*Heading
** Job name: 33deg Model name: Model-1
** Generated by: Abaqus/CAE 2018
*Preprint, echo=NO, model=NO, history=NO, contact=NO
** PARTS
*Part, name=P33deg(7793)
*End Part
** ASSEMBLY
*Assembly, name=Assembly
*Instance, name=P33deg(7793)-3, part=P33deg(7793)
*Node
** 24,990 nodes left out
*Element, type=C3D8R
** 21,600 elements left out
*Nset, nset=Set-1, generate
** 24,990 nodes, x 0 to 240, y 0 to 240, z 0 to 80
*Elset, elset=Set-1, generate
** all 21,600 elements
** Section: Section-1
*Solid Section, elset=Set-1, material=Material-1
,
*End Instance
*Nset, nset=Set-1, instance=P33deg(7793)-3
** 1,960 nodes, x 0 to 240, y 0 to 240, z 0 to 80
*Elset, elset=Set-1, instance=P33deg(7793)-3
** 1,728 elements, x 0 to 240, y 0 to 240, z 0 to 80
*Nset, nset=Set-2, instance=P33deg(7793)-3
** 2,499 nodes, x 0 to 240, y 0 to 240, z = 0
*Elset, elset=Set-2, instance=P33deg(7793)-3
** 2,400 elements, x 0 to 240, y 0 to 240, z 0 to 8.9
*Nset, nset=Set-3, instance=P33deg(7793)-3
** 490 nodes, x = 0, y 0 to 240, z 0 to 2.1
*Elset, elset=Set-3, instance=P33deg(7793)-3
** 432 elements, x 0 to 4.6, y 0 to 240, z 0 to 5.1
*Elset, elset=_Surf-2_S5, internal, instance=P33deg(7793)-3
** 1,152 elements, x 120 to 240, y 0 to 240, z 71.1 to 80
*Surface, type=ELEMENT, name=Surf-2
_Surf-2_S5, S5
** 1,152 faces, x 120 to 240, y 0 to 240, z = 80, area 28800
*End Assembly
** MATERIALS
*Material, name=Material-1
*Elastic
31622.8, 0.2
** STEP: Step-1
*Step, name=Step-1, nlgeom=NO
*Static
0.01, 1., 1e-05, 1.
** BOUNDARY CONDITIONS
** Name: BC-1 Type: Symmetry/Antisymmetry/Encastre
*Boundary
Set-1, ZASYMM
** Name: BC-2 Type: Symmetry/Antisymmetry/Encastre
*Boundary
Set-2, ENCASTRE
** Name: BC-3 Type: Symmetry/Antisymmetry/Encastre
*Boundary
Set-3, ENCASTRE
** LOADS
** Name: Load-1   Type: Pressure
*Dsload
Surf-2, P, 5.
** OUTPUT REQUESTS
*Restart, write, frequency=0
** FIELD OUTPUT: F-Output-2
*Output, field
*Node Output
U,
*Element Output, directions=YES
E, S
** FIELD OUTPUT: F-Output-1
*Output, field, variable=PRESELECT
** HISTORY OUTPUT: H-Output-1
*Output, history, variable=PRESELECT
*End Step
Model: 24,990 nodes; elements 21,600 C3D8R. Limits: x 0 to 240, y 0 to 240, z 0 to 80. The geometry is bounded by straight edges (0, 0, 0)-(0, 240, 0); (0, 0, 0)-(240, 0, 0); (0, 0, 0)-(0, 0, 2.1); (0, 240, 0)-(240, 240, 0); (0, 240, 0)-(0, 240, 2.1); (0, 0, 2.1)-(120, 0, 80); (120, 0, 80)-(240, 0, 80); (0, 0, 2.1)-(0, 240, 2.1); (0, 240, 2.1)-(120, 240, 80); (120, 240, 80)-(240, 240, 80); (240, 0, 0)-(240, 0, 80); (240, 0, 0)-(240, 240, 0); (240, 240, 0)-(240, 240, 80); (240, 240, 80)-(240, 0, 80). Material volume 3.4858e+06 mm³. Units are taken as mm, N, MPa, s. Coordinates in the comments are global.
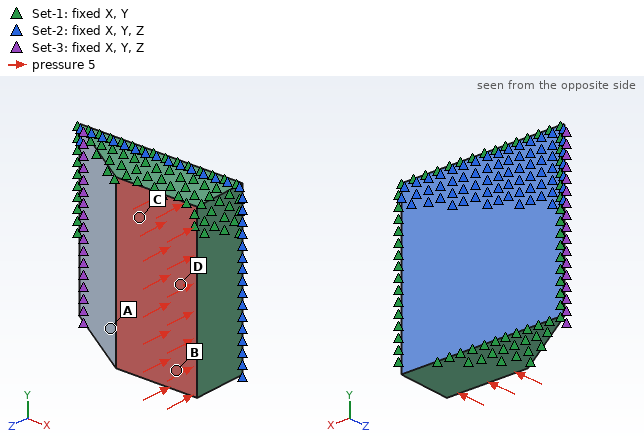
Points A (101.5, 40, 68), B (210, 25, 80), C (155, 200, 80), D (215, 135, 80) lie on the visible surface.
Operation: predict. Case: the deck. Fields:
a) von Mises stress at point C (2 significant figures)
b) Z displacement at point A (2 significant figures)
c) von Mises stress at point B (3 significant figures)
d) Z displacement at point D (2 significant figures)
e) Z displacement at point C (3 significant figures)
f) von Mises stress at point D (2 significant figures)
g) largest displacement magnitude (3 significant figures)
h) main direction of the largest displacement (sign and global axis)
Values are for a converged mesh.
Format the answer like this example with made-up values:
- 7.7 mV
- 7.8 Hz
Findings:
- 3.2 MPa
- -0.0019 mm
- 3.65 MPa
- -0.011 mm
- -0.0105 mm
- 3.6 MPa
- 0.0115 mm
- -Z
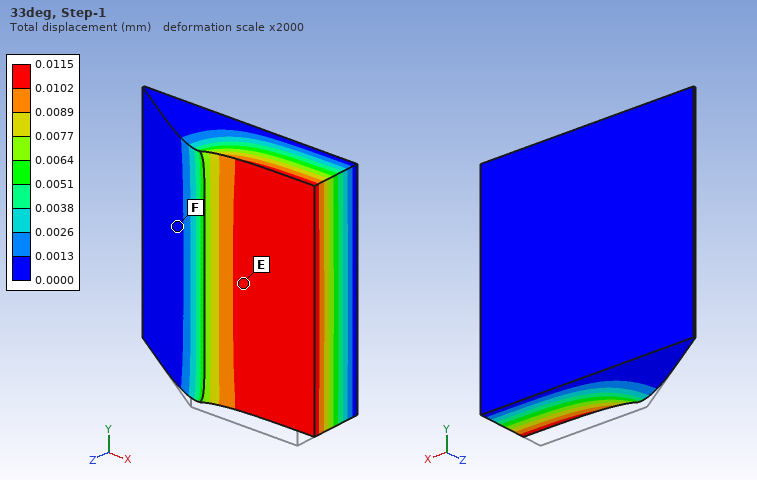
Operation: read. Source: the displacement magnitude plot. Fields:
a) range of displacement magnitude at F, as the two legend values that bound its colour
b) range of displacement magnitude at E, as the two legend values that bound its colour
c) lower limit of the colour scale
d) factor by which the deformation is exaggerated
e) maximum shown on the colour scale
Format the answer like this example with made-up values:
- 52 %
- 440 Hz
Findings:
- 0.0000 to 0.0013 mm
- 0.0102 to 0.0115 mm
- 0.0000 mm
- 2000
- 0.0115 mm
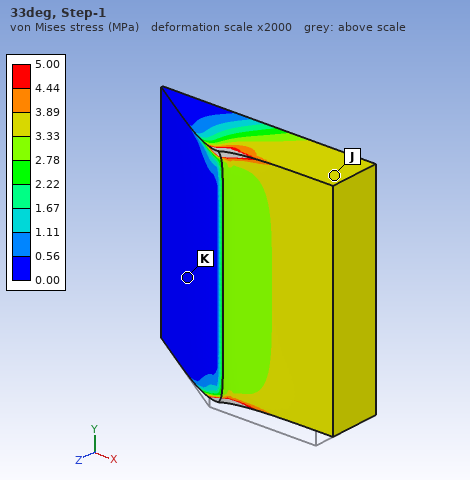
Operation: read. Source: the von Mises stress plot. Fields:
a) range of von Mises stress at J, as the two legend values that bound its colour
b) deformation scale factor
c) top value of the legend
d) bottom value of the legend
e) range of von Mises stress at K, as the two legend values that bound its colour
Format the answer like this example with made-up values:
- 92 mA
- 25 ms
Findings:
- 3.33 to 3.89 MPa
- 2000
- 5.00 MPa
- 0.00 MPa
- 0.00 to 0.56 MPa
